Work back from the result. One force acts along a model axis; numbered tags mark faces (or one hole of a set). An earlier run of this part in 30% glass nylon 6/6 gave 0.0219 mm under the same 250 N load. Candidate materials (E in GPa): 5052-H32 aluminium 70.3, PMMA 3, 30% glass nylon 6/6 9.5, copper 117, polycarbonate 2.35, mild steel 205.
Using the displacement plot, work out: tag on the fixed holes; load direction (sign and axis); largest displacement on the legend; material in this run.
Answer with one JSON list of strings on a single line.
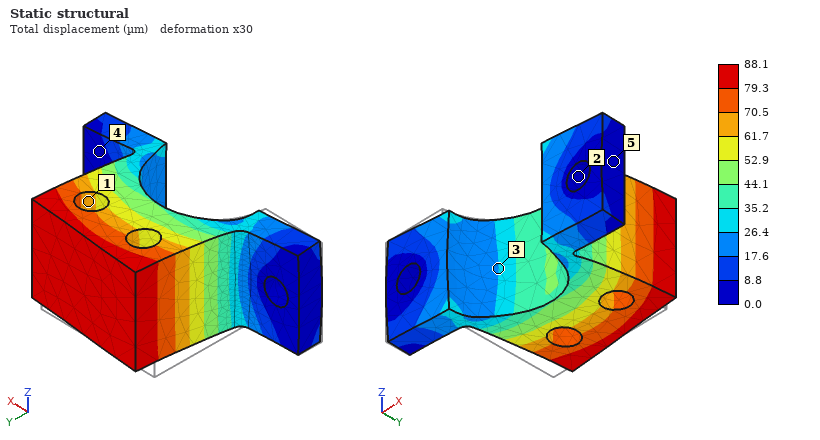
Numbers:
["2", "+X", "88.1 µm", "polycarbonate"]
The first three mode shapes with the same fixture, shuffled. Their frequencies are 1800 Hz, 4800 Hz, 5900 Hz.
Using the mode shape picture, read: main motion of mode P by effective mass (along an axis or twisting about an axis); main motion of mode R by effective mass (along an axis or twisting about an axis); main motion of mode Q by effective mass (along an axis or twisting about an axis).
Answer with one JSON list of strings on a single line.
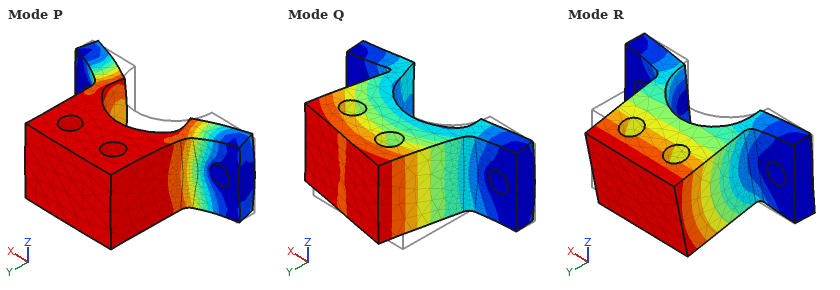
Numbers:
["along Y", "along Z", "along X"]
